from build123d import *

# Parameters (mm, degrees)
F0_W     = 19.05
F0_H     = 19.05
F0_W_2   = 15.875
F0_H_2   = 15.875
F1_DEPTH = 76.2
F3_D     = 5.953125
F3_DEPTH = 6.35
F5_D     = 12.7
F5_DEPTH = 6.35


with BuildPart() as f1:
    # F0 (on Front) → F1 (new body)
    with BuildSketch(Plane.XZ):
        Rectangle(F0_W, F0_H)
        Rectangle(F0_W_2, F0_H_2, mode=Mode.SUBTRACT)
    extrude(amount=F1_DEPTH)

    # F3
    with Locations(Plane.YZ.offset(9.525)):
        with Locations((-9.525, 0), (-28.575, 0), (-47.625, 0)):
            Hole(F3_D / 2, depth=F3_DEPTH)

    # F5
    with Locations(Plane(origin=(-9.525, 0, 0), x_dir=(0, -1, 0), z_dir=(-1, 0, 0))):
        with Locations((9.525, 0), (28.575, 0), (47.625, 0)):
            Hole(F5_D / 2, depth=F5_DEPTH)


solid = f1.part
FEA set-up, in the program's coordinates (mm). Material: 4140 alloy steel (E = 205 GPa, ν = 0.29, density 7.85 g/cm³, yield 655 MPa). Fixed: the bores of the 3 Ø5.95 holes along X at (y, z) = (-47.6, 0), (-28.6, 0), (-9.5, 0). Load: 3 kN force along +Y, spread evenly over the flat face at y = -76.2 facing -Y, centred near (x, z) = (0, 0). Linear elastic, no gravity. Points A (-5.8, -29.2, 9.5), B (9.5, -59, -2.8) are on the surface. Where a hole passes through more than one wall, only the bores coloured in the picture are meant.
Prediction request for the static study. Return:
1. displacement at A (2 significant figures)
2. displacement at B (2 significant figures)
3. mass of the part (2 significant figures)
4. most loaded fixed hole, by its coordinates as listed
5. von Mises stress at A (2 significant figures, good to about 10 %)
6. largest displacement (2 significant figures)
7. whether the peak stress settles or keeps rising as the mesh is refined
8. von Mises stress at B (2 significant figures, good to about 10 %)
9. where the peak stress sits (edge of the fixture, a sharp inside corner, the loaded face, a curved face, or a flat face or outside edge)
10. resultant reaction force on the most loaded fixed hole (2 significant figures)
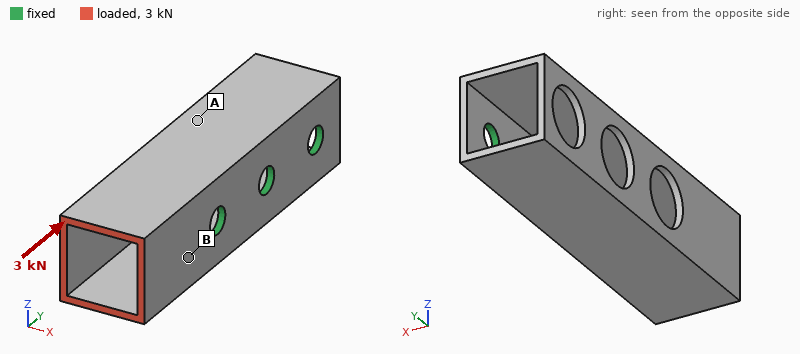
14 µm
19 µm
61 g
(-47.6, 0)
29 MPa
53 µm
keeps rising
76 MPa
edge of the fixture
1.6 kN
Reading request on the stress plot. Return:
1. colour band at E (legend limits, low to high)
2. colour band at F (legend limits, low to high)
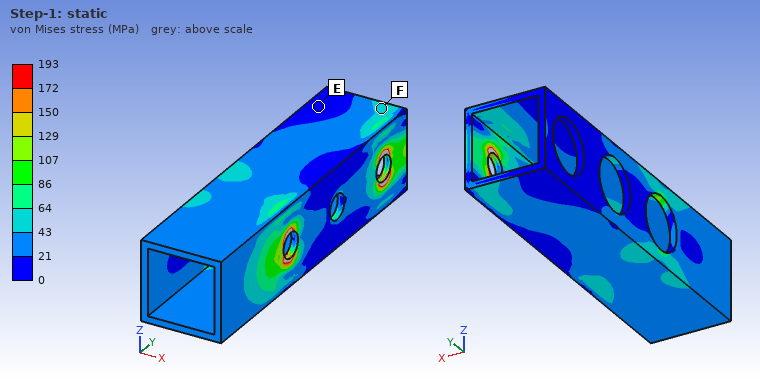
0 to 21 MPa
43 to 64 MPa
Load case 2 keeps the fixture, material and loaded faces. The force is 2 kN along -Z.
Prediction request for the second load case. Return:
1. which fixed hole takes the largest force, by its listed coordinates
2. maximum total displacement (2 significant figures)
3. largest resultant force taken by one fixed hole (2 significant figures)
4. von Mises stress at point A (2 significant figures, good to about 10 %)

(-47.6, 0)
0.27 mm
3.2 kN
82 MPa
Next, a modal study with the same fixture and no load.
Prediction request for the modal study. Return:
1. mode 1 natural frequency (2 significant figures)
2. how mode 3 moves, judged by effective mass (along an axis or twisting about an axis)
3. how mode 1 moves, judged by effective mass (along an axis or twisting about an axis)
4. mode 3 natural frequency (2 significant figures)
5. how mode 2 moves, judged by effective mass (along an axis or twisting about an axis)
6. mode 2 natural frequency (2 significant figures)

2300 Hz
twisting about X
along Z
5900 Hz
along X
4100 Hz
